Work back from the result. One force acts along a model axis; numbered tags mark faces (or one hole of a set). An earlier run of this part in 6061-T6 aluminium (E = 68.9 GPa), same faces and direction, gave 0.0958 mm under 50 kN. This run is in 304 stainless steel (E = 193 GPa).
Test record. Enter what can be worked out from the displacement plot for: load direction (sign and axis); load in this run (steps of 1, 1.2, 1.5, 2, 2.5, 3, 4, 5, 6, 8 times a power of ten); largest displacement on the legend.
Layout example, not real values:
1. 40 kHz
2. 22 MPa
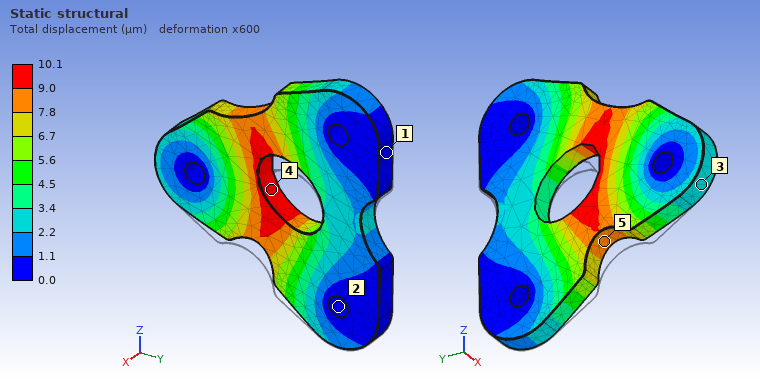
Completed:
1. +Z
2. 15 kN
3. 10.1 µm
